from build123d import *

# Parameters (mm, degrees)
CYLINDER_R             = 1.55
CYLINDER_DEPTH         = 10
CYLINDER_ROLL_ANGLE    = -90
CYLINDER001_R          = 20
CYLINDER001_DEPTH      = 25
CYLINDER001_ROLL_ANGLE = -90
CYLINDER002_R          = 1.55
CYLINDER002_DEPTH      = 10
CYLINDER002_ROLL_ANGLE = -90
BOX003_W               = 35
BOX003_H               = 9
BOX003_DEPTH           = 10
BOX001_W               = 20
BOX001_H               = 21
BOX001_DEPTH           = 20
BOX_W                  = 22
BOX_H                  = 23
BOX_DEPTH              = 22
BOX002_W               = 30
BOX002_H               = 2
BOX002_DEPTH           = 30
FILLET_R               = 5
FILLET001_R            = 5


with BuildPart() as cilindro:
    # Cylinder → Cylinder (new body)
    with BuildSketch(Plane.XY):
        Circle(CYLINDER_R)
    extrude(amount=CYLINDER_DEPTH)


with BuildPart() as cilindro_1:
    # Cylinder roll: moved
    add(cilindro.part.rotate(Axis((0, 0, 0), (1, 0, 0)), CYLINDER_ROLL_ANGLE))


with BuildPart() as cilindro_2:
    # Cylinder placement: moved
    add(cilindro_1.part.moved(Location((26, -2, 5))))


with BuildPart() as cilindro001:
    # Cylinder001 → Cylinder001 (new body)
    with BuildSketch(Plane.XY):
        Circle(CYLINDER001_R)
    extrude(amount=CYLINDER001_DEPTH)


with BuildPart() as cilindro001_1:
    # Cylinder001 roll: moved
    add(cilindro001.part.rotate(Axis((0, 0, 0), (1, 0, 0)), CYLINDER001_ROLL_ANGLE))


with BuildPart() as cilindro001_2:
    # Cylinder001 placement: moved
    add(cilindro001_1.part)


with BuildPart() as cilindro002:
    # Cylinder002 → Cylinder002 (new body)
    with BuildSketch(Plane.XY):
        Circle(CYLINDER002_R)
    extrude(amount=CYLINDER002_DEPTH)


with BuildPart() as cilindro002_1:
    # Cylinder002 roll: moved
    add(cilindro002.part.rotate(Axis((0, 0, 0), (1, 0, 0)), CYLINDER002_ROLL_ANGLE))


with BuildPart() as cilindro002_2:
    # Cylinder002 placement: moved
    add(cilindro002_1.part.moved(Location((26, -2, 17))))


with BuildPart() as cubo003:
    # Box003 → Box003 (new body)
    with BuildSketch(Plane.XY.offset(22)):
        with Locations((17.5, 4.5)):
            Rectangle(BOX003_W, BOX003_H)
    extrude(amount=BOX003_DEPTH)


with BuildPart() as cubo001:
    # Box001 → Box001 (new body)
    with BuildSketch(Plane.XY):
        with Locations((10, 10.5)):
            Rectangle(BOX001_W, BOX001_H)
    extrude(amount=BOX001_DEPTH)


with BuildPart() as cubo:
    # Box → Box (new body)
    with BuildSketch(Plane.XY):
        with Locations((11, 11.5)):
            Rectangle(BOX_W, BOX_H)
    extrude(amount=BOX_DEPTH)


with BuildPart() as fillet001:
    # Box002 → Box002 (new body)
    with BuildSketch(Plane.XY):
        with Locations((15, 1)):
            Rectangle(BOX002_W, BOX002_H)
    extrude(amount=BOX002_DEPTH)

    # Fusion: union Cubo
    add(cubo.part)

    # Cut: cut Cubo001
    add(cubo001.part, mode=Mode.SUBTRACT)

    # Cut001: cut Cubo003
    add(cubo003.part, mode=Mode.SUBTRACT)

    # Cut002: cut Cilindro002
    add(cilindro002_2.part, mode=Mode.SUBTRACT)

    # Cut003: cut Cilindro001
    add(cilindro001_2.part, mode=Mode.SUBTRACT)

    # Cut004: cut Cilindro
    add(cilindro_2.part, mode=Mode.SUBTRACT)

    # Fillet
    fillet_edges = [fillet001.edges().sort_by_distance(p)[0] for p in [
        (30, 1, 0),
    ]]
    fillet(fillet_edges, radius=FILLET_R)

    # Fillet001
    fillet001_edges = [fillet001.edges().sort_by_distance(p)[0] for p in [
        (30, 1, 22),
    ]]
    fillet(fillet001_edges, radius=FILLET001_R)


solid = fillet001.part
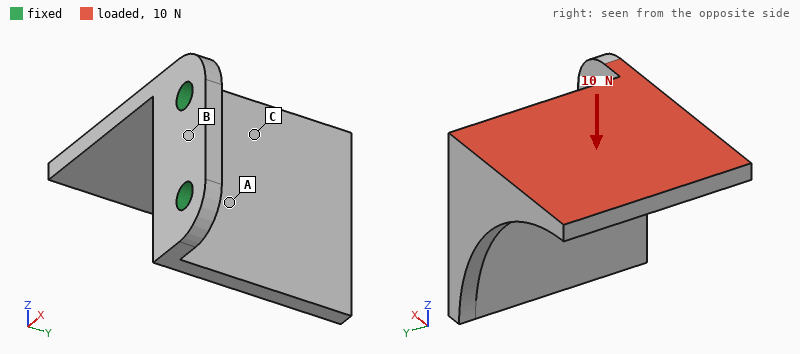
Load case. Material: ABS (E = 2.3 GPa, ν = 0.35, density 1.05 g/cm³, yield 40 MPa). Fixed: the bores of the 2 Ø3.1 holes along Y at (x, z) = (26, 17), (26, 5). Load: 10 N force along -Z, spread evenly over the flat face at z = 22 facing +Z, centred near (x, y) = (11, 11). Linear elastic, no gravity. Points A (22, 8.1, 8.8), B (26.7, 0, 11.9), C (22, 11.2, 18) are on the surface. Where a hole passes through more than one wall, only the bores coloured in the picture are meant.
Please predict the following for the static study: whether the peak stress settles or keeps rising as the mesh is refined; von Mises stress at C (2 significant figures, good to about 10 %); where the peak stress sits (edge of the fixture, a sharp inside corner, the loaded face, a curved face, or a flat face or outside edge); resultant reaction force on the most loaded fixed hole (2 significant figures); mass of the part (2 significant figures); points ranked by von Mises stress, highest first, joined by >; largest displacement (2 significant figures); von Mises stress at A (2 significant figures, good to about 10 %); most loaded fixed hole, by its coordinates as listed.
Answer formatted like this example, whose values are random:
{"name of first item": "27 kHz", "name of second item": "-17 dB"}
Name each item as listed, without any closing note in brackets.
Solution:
{"whether the peak stress settles or keeps rising as the mesh is refined": "keeps rising", "von Mises stress at C": "2.8 MPa", "where the peak stress sits": "a sharp inside corner", "resultant reaction force on the most loaded fixed hole": "14 N", "mass of the part": "2.5 g", "points ranked by von Mises stress, highest first, joined by >": "C > A > B", "largest displacement": "0.44 mm", "von Mises stress at A": "1.7 MPa", "most loaded fixed hole, by its coordinates as listed": "(26, 5)"}
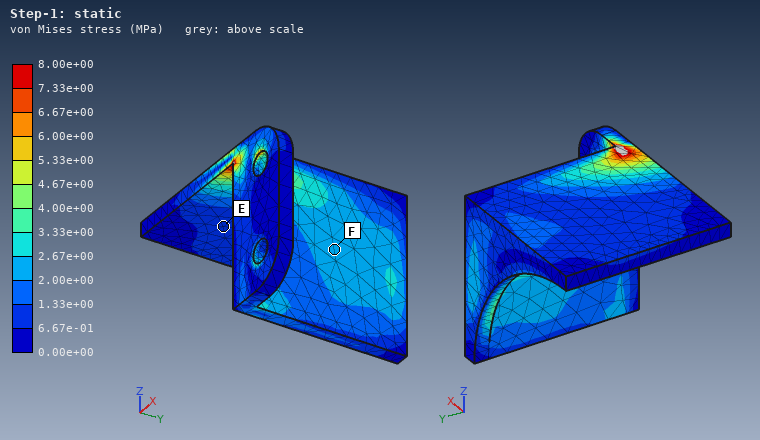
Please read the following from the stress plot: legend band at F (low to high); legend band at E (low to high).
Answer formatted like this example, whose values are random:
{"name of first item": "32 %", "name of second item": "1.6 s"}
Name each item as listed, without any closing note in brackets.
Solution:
{"legend band at F": "2.00e+00 to 2.67e+00 MPa", "legend band at E": "6.67e-01 to 1.33e+00 MPa"}
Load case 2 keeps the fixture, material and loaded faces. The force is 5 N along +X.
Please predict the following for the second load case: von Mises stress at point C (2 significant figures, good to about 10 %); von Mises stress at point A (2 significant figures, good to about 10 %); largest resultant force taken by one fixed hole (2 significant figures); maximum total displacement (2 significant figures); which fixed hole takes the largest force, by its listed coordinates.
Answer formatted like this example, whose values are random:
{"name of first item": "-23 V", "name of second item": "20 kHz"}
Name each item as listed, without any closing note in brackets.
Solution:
{"von Mises stress at point C": "0.65 MPa", "von Mises stress at point A": "1.6 MPa", "largest resultant force taken by one fixed hole": "6.2 N", "maximum total displacement": "0.44 mm", "which fixed hole takes the largest force, by its listed coordinates": "(26, 17)"}
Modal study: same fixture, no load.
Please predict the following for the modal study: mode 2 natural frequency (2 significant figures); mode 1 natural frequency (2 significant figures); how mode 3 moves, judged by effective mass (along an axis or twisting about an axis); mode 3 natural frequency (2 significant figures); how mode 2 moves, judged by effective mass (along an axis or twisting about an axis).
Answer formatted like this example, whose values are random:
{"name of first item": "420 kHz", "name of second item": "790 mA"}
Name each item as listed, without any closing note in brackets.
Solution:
{"mode 2 natural frequency": "870 Hz", "mode 1 natural frequency": "440 Hz", "how mode 3 moves, judged by effective mass": "along Z", "mode 3 natural frequency": "2000 Hz", "how mode 2 moves, judged by effective mass": "along Z"}
